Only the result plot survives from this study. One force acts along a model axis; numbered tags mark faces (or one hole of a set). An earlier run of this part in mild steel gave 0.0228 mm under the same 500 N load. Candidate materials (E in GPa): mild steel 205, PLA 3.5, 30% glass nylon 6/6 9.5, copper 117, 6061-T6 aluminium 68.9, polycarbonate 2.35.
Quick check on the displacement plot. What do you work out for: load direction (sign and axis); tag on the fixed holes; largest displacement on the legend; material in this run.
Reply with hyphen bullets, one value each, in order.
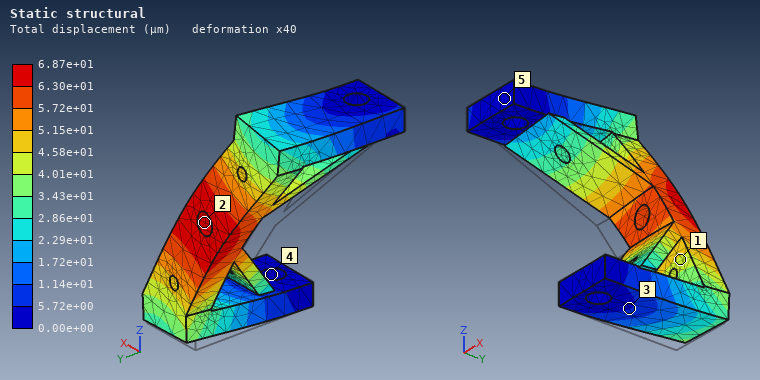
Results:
- +X
- 4
- 6.87e+01 µm
- 6061-T6 aluminium
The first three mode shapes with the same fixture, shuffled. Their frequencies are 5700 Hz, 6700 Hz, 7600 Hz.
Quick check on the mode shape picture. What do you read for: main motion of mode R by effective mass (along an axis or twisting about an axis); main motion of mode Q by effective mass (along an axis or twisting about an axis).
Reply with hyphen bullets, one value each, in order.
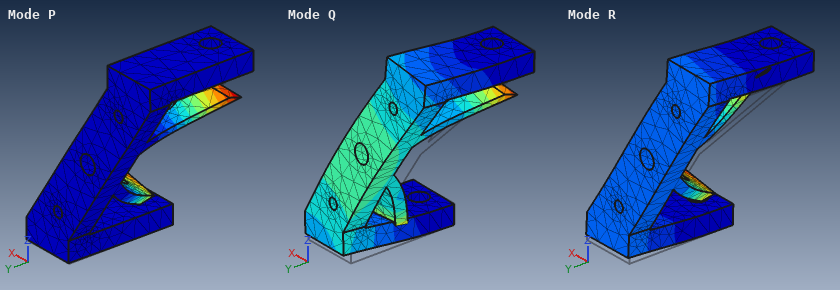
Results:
- along Z
- along X
